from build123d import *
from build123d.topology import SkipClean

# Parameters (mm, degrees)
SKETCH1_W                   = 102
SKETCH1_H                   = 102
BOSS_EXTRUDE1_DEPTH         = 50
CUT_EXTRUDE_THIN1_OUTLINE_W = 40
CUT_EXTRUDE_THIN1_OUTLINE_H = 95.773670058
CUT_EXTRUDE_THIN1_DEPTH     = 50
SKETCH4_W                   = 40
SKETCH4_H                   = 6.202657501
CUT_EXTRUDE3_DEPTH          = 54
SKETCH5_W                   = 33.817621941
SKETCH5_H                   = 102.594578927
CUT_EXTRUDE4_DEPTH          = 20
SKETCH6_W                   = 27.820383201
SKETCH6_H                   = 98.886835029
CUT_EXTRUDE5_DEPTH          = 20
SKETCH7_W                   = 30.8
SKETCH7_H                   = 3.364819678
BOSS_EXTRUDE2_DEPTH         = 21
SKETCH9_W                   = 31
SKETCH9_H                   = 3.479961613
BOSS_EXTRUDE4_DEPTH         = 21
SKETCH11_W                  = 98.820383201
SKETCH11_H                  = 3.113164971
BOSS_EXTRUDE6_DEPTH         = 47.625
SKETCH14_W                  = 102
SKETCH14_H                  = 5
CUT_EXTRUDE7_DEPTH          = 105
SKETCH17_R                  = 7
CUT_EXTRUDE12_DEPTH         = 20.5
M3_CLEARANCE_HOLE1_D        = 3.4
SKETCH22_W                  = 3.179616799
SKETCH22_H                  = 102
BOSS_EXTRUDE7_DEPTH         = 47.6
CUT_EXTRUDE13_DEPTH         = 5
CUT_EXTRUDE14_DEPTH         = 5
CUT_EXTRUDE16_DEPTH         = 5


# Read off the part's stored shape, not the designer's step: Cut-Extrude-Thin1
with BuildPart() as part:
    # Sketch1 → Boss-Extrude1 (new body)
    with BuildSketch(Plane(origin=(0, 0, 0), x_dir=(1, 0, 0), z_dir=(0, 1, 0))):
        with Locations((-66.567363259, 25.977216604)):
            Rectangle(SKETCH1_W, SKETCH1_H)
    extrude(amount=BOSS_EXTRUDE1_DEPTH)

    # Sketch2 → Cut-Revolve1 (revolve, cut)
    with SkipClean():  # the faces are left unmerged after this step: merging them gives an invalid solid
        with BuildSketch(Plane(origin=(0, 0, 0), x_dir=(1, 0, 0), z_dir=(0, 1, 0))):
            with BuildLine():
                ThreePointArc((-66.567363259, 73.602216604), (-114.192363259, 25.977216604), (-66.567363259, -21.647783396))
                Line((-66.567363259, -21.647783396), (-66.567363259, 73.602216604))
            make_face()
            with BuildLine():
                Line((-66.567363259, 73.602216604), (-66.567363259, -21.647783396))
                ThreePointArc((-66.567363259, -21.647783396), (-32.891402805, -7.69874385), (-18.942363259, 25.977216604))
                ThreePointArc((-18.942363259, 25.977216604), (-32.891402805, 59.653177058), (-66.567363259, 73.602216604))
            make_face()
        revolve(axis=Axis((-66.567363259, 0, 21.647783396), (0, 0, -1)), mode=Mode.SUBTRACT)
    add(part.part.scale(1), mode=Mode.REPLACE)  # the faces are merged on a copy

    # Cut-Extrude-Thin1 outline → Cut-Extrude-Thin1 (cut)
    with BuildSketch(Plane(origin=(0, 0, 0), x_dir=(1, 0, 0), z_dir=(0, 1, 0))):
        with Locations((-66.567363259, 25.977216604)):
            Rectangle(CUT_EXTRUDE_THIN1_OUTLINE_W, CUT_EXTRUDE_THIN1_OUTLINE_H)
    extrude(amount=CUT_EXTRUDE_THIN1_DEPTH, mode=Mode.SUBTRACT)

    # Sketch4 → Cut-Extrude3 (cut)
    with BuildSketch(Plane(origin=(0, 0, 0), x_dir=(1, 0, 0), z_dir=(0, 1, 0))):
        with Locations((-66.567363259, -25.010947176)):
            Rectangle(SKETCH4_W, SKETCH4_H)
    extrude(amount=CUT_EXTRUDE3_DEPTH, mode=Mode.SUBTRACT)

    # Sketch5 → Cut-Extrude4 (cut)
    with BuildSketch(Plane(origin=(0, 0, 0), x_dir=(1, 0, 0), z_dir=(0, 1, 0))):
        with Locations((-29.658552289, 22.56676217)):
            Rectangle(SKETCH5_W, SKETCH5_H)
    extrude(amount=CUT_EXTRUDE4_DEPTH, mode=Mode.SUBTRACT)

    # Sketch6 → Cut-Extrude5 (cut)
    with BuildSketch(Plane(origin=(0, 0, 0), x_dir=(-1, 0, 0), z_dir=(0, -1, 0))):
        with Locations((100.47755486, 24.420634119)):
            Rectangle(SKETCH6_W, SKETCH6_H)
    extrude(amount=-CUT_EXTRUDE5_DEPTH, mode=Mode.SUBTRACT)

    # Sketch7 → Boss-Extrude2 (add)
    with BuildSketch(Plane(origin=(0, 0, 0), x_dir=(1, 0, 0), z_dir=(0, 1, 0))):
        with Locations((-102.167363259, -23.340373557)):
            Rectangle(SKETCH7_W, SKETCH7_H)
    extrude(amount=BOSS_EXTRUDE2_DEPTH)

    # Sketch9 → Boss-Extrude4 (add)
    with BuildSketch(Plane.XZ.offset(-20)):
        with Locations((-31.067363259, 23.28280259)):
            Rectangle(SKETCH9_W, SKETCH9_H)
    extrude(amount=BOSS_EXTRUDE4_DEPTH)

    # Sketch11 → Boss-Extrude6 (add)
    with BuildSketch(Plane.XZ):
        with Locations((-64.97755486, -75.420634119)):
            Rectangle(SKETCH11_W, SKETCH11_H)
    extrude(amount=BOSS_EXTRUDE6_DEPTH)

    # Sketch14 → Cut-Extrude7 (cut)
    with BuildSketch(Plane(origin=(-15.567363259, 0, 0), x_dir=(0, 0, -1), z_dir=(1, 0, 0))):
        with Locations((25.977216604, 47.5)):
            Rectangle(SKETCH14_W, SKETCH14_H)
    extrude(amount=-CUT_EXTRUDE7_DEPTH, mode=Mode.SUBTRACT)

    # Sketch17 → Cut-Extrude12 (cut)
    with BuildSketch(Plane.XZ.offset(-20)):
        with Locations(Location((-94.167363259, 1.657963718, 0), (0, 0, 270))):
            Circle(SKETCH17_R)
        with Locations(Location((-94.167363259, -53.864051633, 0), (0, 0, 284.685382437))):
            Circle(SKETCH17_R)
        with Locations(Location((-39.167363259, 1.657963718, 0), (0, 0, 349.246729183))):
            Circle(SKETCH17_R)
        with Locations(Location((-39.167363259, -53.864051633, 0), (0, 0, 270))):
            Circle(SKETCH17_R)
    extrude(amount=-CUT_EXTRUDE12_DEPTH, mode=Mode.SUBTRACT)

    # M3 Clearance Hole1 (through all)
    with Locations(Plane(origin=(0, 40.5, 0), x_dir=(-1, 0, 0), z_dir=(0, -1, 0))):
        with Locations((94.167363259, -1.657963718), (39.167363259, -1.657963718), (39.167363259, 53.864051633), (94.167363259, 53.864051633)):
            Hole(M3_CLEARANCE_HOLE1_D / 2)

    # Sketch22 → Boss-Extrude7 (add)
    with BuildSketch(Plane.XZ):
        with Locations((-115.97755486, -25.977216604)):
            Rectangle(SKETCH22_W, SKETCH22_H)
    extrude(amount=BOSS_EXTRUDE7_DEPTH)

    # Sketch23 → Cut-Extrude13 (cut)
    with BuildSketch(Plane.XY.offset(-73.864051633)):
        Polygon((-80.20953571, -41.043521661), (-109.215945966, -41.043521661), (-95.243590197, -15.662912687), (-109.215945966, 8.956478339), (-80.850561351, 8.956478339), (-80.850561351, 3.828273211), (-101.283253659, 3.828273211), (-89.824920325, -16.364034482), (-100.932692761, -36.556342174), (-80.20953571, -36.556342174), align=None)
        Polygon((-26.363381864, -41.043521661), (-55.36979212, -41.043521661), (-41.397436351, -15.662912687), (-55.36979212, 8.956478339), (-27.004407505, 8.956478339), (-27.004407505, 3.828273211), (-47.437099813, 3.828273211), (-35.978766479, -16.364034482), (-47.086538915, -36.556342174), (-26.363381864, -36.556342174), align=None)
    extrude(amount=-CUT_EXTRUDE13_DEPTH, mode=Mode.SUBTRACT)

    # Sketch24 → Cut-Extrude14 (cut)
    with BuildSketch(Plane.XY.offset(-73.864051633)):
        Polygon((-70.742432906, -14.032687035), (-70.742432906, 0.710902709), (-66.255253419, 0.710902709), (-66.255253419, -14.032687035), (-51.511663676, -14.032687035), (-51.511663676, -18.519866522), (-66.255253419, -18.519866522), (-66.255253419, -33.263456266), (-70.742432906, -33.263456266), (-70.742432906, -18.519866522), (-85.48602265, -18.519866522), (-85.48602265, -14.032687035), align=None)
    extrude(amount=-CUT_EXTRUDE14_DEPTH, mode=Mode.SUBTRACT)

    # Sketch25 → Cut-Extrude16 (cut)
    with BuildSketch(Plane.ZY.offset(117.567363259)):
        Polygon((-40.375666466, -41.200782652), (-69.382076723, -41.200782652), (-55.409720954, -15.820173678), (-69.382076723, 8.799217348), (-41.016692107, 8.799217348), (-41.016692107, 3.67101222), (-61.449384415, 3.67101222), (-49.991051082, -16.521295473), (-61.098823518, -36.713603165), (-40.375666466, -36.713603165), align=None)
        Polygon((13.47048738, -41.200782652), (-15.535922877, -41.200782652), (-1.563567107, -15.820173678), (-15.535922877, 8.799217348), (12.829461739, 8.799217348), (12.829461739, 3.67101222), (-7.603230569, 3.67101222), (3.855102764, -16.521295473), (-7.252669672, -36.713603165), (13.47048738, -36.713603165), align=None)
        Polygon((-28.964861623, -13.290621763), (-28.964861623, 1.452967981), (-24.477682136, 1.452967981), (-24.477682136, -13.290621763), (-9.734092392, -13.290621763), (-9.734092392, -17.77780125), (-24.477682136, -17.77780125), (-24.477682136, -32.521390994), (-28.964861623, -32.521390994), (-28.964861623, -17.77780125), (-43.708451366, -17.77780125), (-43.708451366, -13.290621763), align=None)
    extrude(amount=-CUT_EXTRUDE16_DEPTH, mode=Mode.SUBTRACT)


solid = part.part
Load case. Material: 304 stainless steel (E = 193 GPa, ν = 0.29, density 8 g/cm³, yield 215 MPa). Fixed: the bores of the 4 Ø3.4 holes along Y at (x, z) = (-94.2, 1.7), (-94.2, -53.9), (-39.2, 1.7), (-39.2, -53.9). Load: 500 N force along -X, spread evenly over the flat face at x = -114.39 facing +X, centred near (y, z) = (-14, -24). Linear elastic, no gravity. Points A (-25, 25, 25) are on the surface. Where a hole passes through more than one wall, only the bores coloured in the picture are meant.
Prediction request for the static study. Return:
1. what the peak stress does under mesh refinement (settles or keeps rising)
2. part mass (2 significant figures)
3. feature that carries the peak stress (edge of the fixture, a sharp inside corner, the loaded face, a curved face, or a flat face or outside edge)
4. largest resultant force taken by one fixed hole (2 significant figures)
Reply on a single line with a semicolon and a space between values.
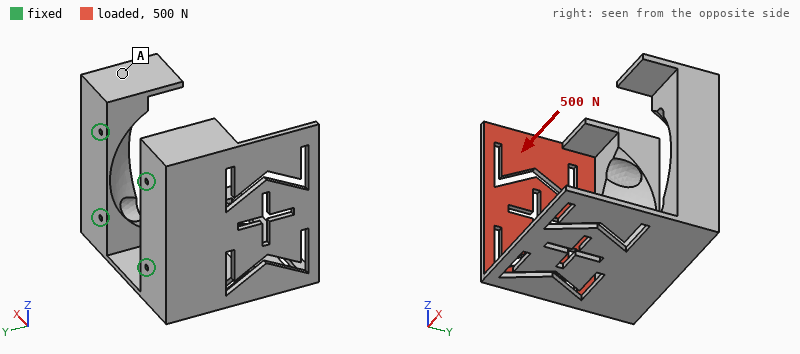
keeps rising; 1.3 kg; edge of the fixture; 530 N
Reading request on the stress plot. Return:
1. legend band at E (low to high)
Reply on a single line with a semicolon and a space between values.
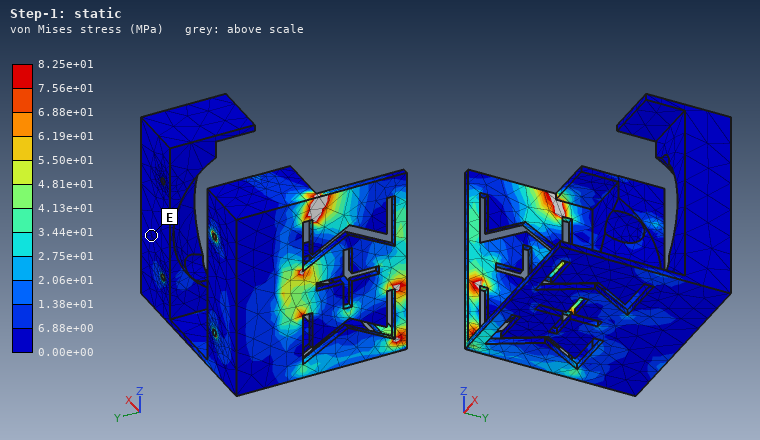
0.00e+00 to 6.88e+00 MPa
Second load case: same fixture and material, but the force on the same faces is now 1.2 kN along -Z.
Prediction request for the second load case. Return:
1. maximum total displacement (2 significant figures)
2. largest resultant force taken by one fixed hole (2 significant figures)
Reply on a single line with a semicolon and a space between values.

83 µm; 1.4 kN
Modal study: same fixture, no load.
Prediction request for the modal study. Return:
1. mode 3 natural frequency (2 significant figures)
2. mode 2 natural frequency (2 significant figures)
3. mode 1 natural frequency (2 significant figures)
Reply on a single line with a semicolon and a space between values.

1100 Hz; 710 Hz; 550 Hz
